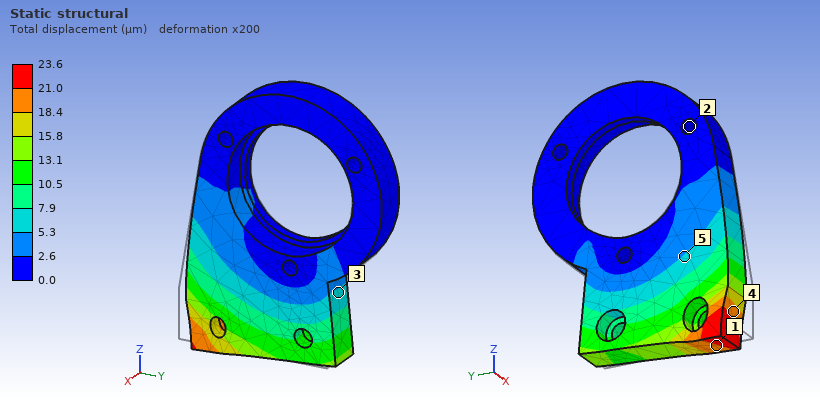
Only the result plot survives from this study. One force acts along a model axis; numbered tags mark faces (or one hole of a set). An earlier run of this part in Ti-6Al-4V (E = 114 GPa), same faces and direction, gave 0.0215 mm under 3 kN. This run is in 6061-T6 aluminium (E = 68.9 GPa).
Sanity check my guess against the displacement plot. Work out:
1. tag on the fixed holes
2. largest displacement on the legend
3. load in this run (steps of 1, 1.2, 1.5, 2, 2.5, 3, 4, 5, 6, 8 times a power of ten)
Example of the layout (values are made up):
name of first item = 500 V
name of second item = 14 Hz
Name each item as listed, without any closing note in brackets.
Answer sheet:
tag on the fixed holes = 2
largest displacement on the legend = 23.6 µm
load in this run = 2 kN
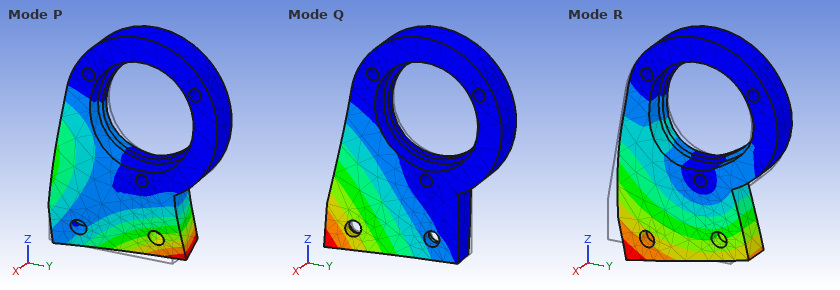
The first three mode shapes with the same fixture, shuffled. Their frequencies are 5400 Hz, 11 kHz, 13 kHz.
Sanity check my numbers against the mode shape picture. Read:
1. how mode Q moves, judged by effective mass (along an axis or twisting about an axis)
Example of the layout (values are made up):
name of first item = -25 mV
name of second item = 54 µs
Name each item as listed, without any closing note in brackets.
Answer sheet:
how mode Q moves, judged by effective mass = along X
